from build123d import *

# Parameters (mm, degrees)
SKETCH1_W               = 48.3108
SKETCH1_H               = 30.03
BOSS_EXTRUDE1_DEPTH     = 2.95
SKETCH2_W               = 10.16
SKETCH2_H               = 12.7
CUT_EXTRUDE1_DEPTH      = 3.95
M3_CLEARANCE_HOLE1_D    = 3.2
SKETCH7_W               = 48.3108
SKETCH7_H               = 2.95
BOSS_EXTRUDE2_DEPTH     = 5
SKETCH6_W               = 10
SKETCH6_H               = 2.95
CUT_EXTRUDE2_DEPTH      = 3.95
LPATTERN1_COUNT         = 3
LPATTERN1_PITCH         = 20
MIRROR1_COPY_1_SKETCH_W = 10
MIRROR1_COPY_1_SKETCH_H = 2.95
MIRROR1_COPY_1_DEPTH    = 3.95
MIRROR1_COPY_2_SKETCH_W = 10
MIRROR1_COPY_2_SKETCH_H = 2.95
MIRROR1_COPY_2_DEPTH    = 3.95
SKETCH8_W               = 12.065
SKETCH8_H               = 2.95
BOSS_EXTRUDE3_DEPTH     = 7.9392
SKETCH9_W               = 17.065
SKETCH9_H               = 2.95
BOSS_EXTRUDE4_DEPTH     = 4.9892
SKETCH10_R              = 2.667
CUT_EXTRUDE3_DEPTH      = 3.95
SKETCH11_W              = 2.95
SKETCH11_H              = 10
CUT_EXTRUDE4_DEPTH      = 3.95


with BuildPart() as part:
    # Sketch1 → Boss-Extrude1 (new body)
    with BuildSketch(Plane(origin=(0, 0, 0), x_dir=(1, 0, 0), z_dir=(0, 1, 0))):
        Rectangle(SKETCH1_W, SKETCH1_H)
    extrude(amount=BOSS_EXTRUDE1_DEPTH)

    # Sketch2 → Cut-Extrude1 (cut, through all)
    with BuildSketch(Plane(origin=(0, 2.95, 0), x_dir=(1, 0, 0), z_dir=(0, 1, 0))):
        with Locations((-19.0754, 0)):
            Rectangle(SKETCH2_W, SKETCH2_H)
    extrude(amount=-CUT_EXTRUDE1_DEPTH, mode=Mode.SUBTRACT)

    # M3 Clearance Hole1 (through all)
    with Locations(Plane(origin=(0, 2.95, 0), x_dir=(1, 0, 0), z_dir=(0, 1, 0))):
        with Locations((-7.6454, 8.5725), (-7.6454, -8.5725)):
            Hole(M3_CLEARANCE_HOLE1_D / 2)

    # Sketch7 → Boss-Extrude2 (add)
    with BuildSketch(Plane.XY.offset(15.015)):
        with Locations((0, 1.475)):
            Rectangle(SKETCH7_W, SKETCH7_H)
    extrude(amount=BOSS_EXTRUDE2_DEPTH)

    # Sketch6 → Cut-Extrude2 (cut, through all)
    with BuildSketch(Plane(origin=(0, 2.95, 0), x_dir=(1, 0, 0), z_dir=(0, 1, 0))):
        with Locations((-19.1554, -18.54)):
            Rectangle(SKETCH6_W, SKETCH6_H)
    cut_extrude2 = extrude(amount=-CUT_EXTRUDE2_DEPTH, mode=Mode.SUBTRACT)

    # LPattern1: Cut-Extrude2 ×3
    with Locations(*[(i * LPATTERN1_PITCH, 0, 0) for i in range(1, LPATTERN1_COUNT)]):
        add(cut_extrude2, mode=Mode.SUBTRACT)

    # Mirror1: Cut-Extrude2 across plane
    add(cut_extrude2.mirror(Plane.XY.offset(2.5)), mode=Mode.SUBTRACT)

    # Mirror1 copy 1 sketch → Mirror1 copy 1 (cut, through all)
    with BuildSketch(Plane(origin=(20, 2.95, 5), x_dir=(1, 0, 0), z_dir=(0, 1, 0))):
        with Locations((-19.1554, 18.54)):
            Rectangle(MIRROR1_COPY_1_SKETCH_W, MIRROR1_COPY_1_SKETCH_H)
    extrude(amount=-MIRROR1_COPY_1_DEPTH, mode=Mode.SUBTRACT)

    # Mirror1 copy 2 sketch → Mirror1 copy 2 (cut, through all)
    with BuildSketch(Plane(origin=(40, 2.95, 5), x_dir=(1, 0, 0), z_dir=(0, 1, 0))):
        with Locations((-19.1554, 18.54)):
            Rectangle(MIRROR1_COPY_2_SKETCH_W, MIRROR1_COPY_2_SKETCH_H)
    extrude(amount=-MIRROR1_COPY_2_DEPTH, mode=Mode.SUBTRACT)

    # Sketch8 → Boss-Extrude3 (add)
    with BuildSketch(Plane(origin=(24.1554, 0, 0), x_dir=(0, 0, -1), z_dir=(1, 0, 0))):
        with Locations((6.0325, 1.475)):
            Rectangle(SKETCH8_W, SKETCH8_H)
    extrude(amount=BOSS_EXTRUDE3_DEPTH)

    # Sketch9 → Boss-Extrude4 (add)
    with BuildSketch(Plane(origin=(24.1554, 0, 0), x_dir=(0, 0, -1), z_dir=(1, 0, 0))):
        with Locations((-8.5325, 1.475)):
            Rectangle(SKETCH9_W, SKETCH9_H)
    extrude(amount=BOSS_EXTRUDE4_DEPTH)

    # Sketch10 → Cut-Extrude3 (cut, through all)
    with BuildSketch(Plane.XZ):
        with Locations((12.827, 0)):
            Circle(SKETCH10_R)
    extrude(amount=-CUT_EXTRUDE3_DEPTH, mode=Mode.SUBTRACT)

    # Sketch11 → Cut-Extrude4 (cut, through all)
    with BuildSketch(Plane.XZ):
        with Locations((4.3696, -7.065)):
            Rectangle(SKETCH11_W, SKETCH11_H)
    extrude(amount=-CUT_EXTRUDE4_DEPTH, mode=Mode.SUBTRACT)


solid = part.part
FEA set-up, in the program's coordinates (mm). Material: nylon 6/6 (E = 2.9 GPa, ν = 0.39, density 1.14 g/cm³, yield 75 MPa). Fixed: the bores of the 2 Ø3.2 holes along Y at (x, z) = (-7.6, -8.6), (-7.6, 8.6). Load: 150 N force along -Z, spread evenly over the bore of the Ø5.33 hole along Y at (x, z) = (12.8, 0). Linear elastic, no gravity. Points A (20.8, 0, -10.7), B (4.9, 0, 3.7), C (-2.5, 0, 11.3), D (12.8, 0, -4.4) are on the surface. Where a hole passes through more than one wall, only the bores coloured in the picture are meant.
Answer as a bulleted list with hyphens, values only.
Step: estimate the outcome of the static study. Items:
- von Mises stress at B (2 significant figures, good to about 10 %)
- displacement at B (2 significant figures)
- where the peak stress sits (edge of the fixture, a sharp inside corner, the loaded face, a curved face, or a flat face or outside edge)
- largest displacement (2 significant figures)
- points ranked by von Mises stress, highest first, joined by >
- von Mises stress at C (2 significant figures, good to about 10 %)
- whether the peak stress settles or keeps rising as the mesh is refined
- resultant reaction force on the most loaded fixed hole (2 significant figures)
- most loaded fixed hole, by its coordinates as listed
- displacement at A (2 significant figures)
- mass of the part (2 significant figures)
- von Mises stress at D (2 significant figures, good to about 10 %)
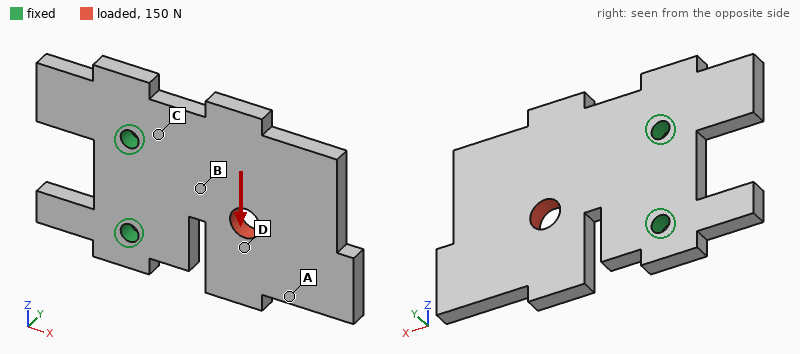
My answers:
- 7.8 MPa
- 0.058 mm
- a sharp inside corner
- 0.28 mm
- B > C > D > A
- 5.0 MPa
- keeps rising
- 190 N
- (-7.6, -8.6)
- 0.22 mm
- 5.1 g
- 2.7 MPa
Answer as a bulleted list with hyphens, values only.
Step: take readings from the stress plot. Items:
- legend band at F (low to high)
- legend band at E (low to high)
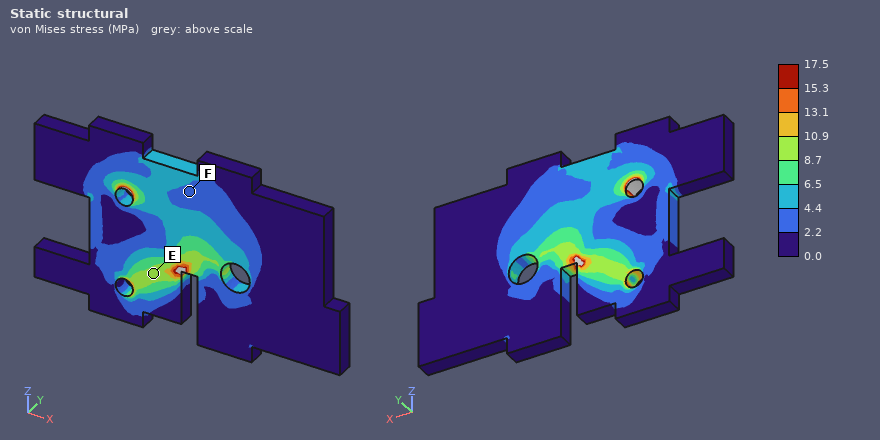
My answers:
- 2.2 to 4.4 MPa
- 8.7 to 10.9 MPa
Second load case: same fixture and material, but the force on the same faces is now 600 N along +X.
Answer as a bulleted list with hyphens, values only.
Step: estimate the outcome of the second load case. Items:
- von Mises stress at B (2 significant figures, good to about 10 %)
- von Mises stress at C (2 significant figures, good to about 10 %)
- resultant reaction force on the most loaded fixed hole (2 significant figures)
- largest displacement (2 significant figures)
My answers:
- 13 MPa
- 5.4 MPa
- 330 N
- 0.56 mm
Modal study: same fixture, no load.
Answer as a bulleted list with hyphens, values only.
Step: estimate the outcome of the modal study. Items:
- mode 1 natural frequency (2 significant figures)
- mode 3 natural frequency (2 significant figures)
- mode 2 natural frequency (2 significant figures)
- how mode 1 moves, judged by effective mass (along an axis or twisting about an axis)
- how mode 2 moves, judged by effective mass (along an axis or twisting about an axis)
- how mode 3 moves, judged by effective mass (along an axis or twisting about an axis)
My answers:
- 460 Hz
- 2200 Hz
- 1100 Hz
- along Y
- twisting about X
- along Z
